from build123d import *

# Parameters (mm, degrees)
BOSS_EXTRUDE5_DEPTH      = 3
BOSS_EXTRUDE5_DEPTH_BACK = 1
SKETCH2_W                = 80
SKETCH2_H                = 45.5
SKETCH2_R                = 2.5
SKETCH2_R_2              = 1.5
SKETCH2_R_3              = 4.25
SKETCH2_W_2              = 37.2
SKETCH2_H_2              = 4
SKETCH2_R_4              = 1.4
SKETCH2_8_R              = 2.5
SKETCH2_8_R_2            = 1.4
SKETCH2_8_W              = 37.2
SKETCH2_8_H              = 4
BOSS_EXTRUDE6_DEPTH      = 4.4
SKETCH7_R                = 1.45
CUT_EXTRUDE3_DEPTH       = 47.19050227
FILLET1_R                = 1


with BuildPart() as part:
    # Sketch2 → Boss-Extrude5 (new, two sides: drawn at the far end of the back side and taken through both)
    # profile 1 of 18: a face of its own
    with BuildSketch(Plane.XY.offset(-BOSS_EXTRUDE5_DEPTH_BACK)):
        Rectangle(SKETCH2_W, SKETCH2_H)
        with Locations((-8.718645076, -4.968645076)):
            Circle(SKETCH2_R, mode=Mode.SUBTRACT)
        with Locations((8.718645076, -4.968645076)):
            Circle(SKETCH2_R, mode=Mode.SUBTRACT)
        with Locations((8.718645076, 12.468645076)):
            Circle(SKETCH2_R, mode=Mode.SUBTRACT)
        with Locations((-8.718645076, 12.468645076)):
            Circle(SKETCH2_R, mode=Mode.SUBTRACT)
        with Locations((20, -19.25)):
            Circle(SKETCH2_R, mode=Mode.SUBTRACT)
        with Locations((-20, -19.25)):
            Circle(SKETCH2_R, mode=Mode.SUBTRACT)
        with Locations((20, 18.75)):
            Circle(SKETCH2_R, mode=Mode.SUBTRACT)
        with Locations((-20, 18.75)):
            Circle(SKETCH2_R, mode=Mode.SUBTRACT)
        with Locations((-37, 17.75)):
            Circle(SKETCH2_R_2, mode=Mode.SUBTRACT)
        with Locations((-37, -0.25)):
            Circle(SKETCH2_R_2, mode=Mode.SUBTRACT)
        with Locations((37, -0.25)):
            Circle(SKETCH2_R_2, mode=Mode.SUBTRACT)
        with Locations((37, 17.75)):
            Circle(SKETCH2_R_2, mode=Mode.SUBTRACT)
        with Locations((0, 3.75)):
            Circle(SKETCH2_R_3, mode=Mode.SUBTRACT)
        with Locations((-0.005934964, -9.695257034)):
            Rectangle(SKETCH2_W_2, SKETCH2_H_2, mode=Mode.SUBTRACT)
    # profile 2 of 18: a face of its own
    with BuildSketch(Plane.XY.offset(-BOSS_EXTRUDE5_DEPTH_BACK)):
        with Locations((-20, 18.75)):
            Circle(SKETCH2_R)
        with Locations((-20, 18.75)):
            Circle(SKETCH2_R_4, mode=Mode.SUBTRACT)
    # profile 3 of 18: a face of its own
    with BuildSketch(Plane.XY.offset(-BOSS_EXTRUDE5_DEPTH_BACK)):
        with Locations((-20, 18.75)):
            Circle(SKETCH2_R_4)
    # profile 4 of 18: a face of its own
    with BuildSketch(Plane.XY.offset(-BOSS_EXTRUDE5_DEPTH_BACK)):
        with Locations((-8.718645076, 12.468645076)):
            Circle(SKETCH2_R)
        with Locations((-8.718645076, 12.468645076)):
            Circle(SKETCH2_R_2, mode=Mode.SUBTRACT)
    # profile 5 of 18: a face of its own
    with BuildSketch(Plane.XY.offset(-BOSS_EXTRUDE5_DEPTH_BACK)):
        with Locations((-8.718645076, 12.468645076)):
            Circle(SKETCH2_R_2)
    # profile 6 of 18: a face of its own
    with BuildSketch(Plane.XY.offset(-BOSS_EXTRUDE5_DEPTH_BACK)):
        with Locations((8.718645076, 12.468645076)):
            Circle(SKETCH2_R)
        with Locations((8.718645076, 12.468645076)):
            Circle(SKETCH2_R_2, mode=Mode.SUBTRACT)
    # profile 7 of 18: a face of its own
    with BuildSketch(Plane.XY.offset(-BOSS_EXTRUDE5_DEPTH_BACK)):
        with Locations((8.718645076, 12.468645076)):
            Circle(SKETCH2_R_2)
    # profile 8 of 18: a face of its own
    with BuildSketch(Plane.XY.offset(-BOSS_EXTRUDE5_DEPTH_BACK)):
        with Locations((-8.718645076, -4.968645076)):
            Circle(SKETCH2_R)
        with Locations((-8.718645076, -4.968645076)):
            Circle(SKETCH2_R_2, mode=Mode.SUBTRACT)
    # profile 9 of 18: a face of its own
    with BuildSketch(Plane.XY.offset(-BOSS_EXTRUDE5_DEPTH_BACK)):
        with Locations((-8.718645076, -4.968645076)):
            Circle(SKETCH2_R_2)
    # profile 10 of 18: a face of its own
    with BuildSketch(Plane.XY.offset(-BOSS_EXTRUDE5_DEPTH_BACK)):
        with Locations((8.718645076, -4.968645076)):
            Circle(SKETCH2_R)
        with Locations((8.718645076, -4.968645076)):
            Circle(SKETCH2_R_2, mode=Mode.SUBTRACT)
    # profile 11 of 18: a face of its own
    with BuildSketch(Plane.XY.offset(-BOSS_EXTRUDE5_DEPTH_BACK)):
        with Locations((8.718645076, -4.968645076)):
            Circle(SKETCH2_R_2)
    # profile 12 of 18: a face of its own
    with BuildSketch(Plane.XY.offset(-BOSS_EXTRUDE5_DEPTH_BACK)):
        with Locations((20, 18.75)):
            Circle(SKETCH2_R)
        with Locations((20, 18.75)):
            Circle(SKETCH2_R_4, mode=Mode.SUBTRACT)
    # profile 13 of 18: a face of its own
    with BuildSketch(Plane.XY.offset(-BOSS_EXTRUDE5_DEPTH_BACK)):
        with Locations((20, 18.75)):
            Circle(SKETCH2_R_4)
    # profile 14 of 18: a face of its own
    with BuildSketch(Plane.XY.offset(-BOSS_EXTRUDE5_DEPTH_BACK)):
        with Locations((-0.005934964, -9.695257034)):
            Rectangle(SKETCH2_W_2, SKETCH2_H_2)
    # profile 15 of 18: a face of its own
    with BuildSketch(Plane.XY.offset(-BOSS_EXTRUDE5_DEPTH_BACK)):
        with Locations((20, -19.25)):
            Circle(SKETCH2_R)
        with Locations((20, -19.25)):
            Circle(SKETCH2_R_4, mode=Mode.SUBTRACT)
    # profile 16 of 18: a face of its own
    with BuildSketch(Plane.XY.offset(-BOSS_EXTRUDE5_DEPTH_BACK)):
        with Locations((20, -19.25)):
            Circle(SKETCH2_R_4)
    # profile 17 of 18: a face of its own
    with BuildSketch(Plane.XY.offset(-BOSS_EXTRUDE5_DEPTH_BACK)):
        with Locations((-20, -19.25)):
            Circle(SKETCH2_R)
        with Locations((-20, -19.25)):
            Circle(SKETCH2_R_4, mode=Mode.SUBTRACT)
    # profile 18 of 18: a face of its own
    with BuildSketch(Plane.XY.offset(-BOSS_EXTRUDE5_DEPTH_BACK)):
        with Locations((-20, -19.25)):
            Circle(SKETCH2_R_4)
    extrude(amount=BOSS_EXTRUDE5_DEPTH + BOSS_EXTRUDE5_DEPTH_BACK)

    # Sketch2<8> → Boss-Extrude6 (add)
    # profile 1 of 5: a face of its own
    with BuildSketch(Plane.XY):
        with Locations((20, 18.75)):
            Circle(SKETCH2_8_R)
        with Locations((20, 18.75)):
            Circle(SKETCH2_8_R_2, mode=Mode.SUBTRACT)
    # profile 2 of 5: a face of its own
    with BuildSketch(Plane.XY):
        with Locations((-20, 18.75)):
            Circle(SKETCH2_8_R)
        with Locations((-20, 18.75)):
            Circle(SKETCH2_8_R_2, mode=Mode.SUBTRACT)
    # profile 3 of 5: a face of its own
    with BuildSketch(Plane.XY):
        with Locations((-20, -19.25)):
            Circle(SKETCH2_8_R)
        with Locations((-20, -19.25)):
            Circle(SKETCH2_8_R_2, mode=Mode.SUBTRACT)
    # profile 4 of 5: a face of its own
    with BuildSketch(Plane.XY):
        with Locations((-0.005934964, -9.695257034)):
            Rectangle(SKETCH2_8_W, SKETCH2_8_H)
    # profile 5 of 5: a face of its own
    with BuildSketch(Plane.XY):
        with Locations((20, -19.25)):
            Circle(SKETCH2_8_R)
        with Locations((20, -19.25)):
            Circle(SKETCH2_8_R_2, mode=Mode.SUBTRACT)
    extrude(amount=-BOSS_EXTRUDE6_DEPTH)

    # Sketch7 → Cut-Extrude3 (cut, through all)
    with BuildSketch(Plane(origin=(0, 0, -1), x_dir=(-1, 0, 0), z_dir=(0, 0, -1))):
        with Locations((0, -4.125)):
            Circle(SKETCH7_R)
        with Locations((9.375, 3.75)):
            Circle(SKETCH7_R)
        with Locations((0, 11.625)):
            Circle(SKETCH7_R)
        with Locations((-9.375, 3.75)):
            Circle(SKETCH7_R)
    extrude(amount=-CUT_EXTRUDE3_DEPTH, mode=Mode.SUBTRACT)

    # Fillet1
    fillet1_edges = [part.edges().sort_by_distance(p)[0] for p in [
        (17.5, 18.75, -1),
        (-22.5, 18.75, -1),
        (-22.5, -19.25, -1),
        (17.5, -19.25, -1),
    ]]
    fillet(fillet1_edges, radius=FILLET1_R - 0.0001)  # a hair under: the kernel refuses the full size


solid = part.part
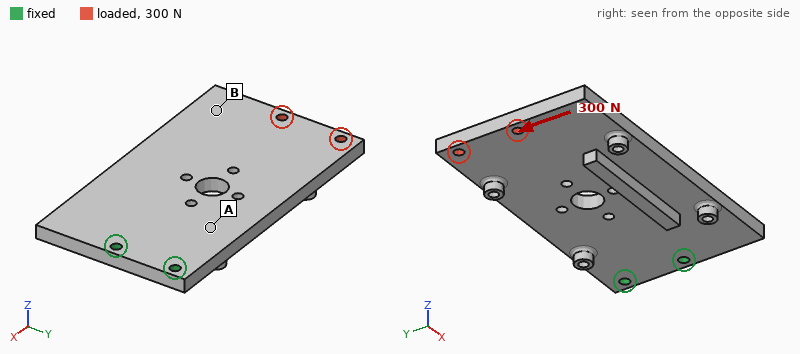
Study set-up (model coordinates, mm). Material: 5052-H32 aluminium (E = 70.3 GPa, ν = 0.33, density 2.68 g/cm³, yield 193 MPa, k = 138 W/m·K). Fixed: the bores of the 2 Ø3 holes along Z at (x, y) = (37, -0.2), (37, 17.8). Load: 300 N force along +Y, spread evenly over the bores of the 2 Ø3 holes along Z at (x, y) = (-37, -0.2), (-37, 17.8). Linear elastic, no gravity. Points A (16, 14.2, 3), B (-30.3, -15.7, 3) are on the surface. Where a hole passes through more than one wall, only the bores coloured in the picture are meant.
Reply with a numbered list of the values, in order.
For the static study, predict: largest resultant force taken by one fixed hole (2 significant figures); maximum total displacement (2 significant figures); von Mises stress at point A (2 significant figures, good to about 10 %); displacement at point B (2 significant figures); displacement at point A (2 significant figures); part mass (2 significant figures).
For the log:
1. 1.2 kN
2. 66 µm
3. 10.0 MPa
4. 56 µm
5. 13 µm
6. 40 g
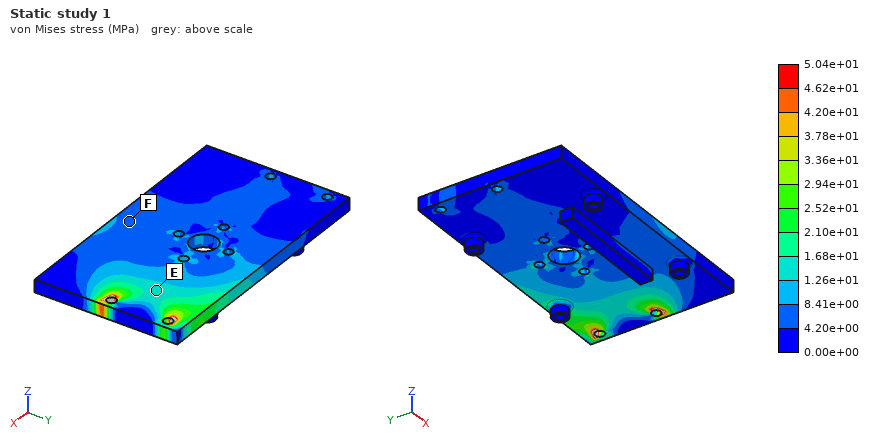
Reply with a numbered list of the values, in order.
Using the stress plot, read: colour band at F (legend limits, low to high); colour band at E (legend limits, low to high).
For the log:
1. 4.20e+00 to 8.41e+00 MPa
2. 1.26e+01 to 1.68e+01 MPa
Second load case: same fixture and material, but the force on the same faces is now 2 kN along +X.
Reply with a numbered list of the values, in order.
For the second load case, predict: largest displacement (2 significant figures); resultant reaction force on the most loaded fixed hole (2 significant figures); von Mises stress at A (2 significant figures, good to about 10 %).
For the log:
1. 36 µm
2. 1.0 kN
3. 20 MPa
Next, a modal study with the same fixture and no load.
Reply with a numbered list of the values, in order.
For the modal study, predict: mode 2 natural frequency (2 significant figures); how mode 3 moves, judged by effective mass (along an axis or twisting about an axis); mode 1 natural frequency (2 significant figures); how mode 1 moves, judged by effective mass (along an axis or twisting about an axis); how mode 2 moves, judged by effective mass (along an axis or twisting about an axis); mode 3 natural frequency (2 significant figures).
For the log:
1. 1800 Hz
2. along Y
3. 520 Hz
4. along Z
5. twisting about X
6. 3000 Hz
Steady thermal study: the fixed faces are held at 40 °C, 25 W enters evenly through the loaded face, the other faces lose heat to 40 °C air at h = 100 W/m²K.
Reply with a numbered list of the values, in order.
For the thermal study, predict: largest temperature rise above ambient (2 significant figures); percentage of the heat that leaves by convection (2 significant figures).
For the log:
1. 57 K
2. 67 %
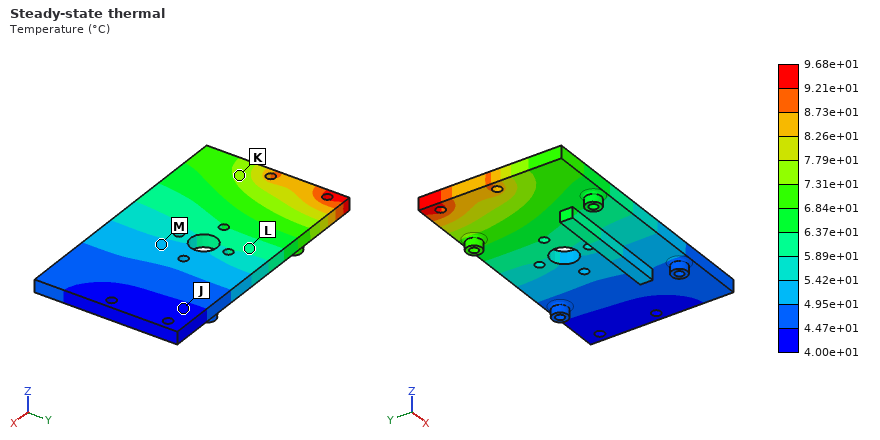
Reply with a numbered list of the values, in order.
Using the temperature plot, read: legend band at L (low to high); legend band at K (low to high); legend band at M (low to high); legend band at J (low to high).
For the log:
1. 5.89e+01 to 6.37e+01 °C
2. 7.31e+01 to 7.79e+01 °C
3. 4.95e+01 to 5.42e+01 °C
4. 4.00e+01 to 4.47e+01 °C
